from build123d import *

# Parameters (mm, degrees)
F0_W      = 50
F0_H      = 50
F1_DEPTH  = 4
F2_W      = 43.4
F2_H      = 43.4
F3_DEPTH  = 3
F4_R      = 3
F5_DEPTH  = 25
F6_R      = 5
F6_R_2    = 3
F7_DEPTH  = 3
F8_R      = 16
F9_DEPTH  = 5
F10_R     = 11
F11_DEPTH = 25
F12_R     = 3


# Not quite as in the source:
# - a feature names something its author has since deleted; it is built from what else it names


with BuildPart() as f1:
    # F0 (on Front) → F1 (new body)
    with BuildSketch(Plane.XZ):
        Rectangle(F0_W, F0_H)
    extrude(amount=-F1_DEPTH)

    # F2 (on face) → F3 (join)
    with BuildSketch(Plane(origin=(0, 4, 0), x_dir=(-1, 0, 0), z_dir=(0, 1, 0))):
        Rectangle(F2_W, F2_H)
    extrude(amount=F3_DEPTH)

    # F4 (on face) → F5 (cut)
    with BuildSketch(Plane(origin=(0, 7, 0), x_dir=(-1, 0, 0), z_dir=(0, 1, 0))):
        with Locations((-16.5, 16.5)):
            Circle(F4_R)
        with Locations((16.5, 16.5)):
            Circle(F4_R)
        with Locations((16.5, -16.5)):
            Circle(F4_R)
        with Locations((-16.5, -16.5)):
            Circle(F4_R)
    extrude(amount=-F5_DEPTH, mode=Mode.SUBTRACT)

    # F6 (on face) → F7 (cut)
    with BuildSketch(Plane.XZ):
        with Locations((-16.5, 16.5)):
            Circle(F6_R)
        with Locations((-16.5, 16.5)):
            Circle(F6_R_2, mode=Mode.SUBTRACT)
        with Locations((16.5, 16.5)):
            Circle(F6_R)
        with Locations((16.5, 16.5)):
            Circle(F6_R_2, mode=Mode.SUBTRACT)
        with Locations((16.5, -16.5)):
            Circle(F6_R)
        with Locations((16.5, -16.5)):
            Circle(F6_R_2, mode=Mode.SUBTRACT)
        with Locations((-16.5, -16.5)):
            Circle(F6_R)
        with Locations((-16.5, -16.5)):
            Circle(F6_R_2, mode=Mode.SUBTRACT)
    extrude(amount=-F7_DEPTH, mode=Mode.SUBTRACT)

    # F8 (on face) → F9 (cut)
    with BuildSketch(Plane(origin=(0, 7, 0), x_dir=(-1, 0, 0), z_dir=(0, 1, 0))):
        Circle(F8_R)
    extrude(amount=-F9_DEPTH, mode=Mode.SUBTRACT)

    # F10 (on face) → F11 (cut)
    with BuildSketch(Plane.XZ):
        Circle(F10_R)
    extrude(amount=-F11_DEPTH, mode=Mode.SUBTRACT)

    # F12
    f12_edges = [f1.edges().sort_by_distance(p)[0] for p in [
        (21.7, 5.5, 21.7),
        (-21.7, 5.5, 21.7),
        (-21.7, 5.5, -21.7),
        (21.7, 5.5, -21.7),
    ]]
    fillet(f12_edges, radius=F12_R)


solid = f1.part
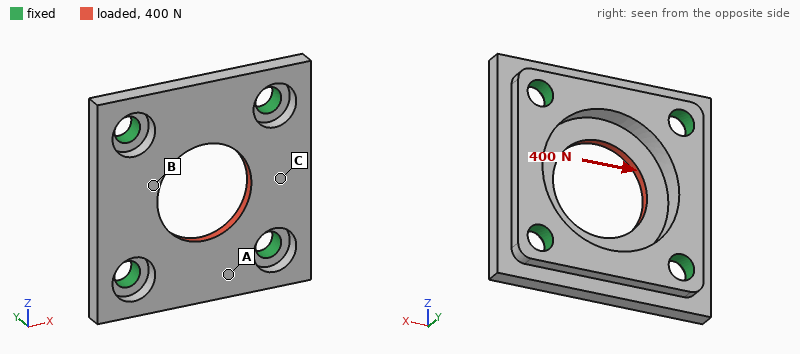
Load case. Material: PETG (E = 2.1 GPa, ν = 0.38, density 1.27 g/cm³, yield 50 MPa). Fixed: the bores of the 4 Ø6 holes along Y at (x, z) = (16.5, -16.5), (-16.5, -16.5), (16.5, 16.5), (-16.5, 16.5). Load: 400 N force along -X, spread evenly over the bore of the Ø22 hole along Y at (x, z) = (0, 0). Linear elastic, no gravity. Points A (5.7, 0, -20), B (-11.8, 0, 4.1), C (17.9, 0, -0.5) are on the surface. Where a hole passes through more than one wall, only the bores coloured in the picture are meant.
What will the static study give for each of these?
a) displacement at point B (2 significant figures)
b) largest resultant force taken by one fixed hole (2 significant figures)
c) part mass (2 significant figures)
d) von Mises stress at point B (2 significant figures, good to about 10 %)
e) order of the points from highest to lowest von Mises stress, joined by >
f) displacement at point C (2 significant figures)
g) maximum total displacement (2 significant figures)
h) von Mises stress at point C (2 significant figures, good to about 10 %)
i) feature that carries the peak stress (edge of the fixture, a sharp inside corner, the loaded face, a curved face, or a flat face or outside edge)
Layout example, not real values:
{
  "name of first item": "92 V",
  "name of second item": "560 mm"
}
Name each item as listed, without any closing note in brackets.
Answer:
{
  "displacement at point B": "44 µm",
  "largest resultant force taken by one fixed hole": "100 N",
  "part mass": "12 g",
  "von Mises stress at point B": "3.1 MPa",
  "order of the points from highest to lowest von Mises stress, joined by >": "B > C > A",
  "displacement at point C": "34 µm",
  "maximum total displacement": "52 µm",
  "von Mises stress at point C": "1.8 MPa",
  "feature that carries the peak stress": "edge of the fixture"
}
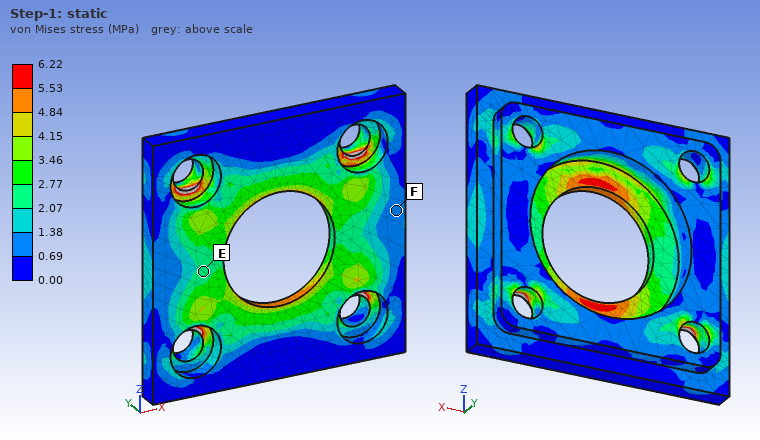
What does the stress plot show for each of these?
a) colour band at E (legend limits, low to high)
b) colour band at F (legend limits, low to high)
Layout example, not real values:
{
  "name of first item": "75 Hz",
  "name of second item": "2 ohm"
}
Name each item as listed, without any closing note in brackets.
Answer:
{
  "colour band at E": "2.07 to 2.77 MPa",
  "colour band at F": "0.69 to 1.38 MPa"
}
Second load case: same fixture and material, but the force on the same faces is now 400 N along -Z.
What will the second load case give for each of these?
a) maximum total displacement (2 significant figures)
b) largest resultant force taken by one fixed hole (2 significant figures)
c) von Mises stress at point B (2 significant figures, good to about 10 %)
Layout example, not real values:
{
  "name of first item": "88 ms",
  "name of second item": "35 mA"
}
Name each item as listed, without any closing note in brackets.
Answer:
{
  "maximum total displacement": "52 µm",
  "largest resultant force taken by one fixed hole": "100 N",
  "von Mises stress at point B": "3.3 MPa"
}
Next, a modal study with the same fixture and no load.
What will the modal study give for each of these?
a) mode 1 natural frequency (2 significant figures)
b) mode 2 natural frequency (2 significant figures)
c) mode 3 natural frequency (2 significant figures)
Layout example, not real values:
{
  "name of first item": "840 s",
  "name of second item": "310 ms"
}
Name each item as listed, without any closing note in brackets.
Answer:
{
  "mode 1 natural frequency": "5800 Hz",
  "mode 2 natural frequency": "6400 Hz",
  "mode 3 natural frequency": "6400 Hz"
}
